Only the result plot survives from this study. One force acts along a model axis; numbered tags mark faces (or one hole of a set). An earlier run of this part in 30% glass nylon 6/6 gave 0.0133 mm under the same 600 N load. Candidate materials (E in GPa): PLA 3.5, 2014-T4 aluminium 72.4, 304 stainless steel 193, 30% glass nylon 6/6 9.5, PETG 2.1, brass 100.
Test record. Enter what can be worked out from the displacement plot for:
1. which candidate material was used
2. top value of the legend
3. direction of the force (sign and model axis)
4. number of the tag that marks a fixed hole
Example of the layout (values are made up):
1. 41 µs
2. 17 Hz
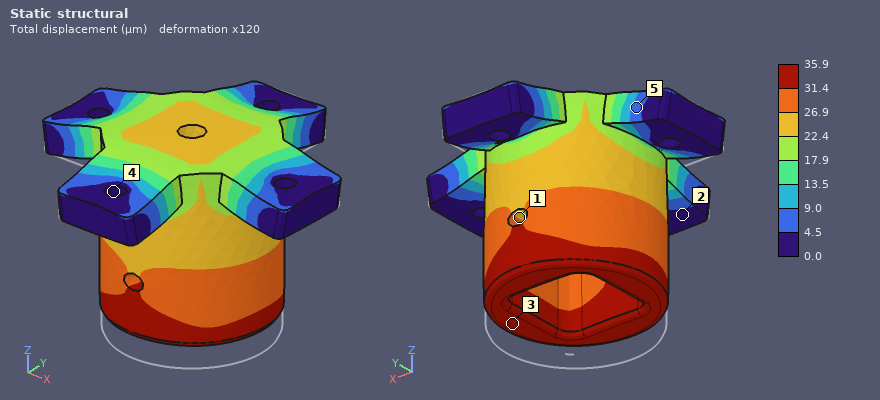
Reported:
1. PLA
2. 35.9 µm
3. +Z
4. 4
